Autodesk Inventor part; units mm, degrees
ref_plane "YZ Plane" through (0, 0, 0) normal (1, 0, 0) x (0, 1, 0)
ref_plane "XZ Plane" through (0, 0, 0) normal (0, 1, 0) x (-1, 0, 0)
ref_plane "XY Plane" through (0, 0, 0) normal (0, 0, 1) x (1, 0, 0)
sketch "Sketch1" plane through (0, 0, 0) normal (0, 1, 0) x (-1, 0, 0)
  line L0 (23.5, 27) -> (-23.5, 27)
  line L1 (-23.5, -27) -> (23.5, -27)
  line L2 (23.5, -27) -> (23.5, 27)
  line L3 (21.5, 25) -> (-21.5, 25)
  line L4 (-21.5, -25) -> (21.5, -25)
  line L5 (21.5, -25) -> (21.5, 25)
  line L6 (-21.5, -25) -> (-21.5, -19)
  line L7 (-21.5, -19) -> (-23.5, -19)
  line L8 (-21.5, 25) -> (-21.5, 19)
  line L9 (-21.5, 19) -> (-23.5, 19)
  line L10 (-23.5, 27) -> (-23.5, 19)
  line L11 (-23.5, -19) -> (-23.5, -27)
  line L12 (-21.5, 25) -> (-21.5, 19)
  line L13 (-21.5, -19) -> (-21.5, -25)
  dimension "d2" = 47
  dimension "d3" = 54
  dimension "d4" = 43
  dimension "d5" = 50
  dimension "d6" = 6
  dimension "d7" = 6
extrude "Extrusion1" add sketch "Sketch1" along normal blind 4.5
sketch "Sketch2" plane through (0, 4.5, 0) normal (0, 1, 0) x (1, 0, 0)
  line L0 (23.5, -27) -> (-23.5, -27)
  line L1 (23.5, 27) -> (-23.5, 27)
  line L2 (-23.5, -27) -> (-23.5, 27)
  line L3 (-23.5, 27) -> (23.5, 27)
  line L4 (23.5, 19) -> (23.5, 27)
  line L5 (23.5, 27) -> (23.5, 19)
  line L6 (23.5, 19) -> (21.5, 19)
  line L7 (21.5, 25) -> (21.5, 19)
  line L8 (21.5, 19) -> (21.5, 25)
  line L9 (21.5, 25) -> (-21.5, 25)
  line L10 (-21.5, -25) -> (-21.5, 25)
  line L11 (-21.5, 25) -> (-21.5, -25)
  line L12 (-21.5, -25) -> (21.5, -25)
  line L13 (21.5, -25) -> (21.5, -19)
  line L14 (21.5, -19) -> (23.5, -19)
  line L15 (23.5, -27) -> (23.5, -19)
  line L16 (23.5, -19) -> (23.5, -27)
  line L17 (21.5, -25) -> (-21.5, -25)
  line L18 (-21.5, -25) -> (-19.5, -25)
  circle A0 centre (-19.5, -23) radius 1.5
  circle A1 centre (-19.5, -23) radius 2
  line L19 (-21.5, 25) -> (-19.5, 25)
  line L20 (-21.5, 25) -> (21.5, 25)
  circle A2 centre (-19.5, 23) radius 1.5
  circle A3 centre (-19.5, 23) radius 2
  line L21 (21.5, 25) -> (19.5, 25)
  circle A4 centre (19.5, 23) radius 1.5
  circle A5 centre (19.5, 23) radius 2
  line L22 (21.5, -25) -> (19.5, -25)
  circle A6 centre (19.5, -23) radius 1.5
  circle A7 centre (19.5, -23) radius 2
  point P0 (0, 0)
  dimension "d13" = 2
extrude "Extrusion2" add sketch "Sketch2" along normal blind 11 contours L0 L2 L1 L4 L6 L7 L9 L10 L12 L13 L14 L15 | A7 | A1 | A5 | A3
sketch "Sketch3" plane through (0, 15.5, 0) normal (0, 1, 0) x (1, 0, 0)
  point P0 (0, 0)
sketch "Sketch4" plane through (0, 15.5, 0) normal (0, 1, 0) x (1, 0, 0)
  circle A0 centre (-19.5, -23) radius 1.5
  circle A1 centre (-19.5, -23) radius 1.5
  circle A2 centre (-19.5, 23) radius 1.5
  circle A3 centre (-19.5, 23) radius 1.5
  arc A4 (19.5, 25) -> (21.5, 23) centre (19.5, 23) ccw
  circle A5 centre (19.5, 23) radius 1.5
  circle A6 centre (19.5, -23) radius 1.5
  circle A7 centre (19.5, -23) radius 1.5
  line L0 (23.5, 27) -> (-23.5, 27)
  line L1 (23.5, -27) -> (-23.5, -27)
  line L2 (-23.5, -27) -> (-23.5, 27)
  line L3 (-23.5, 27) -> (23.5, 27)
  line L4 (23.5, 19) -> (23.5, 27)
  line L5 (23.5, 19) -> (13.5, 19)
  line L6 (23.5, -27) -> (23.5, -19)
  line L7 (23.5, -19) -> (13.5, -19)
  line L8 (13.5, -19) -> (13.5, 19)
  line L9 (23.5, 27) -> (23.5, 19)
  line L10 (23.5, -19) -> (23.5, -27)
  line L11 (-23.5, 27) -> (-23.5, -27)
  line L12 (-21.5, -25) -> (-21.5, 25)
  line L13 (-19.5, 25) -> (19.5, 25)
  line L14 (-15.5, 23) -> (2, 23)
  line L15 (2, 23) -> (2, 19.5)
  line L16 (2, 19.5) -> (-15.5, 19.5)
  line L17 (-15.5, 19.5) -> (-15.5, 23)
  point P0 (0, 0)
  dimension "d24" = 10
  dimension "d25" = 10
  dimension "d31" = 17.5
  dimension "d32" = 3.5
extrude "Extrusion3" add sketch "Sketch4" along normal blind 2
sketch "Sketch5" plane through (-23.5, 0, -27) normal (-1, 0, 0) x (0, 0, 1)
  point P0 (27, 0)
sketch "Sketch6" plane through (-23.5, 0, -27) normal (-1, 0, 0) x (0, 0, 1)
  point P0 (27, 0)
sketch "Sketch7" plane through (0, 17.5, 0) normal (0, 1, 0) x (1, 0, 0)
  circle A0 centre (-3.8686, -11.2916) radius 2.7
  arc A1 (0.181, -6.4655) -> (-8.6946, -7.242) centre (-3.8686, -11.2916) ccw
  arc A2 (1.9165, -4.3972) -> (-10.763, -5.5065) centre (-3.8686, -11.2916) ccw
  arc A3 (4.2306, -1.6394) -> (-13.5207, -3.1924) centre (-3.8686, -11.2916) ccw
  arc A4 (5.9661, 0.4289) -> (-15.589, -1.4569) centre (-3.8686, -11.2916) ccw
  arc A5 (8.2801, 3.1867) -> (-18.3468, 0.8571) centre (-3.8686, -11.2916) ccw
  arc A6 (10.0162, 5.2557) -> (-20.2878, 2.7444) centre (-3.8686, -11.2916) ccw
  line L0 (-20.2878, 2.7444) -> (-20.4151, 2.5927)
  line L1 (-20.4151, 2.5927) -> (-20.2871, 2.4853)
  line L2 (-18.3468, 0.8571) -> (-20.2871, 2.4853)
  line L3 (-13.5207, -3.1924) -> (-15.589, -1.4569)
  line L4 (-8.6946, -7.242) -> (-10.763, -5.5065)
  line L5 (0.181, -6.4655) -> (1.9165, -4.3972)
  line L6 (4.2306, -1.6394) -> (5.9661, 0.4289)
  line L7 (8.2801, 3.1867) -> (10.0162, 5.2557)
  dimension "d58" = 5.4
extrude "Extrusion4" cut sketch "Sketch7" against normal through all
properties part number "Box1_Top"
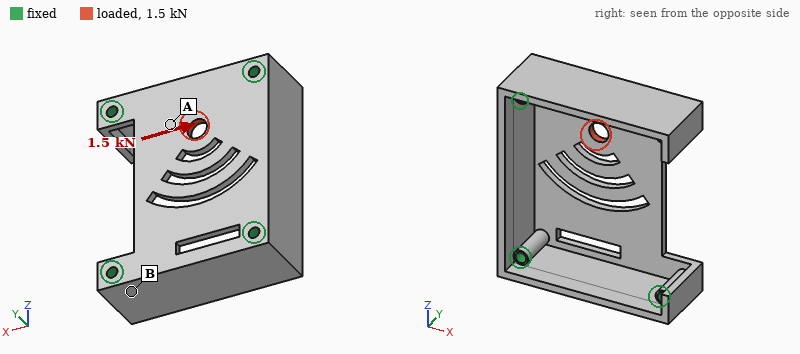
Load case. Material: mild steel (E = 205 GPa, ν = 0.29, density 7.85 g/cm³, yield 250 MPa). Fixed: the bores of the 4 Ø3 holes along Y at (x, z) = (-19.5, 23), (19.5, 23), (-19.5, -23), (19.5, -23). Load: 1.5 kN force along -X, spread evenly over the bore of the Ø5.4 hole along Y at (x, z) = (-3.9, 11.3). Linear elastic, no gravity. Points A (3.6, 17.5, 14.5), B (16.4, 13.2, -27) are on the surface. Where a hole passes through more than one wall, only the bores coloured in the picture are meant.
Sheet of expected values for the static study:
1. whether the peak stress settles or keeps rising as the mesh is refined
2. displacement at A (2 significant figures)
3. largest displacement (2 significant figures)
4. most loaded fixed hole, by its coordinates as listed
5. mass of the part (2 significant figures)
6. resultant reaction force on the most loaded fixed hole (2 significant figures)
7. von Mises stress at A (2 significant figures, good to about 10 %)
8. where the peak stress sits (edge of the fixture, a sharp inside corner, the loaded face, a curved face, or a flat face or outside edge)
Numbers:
keeps rising
3.5 µm
5.9 µm
(-19.5, 23)
69 g
870 N
37 MPa
edge of the fixture
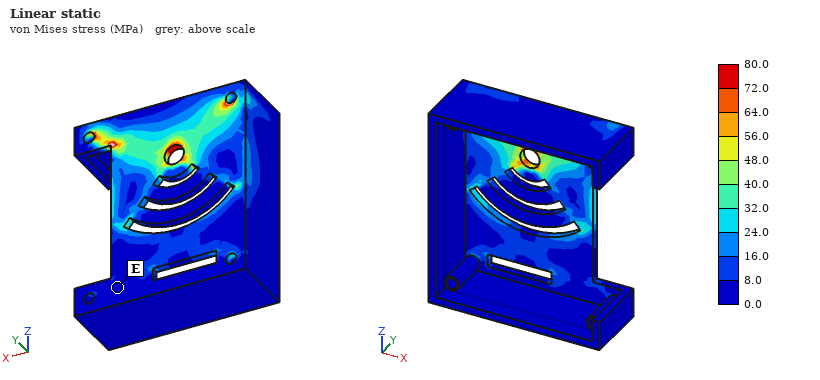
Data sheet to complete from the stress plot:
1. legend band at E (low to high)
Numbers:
0.0 to 8.0 MPa
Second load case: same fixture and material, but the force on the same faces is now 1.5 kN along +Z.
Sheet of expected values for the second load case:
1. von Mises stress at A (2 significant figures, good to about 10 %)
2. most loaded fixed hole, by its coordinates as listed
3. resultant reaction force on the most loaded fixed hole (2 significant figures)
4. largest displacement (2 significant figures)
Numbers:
33 MPa
(-19.5, 23)
870 N
7.9 µm
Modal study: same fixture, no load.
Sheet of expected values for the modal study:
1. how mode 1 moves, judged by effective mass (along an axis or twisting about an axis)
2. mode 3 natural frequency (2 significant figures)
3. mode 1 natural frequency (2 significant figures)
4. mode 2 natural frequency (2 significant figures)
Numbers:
along Y
7600 Hz
4000 Hz
6800 Hz
